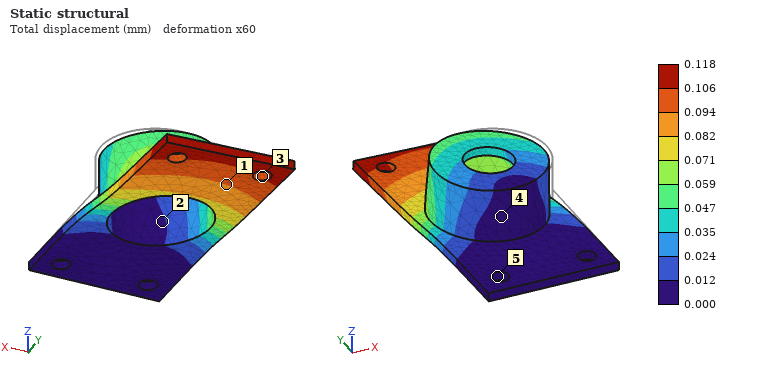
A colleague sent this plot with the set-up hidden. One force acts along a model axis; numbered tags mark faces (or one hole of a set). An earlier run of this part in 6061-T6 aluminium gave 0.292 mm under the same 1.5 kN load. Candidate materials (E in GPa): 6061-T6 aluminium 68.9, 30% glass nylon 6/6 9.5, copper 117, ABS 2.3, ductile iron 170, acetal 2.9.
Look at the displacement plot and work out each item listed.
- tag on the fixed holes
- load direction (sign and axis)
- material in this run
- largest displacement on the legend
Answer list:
5
-X
ductile iron
0.118 mm
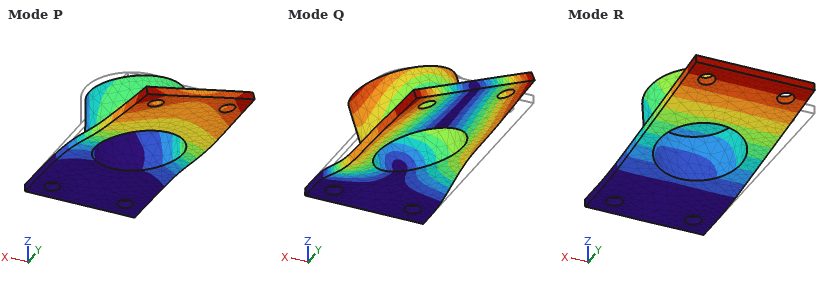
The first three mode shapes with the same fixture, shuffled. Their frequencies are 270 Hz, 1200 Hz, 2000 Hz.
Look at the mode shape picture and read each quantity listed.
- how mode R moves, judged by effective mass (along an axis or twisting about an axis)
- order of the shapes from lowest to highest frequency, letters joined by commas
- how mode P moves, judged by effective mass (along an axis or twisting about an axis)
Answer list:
along Z
R, Q, P
along X
